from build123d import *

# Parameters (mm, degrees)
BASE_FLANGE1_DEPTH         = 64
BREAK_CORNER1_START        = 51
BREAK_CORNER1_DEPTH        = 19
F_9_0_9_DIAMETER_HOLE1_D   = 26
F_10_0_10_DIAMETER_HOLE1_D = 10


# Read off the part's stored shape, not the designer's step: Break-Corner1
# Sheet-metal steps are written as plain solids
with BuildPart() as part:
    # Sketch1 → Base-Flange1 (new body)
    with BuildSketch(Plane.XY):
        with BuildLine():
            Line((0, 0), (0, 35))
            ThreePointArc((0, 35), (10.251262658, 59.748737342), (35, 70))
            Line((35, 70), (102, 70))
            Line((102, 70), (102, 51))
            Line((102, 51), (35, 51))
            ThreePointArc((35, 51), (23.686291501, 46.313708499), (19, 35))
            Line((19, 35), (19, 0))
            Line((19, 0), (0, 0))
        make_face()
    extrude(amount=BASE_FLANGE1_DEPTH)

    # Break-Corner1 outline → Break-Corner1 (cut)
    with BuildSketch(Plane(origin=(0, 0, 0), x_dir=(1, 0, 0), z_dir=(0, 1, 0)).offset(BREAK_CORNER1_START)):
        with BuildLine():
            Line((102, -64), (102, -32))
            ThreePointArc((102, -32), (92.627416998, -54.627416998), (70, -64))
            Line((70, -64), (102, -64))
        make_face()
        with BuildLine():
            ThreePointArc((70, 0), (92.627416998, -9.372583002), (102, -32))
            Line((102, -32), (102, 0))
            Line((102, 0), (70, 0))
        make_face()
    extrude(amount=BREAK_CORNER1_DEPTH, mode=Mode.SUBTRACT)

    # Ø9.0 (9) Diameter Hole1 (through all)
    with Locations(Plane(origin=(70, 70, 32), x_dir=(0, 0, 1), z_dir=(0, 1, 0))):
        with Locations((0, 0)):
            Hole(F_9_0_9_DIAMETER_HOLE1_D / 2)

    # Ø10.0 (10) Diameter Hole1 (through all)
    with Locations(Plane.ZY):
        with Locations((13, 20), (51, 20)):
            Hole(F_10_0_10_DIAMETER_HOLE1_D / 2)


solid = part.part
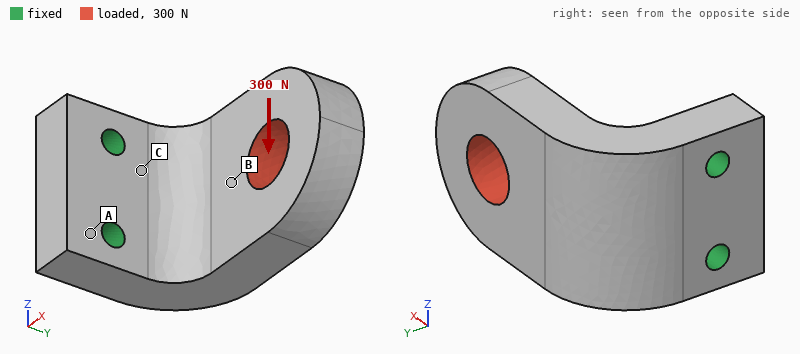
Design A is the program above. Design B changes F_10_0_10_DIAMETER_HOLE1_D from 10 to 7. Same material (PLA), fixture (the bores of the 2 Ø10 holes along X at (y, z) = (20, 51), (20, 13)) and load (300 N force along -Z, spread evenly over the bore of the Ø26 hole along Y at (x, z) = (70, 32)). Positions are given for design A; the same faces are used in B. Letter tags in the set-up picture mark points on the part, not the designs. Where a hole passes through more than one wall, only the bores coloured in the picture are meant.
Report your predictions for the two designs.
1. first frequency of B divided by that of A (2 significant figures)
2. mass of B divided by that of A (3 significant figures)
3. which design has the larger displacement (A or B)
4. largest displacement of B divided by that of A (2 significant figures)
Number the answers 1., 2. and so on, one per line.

1. 0.96
2. 1.01
3. B
4. 1.1
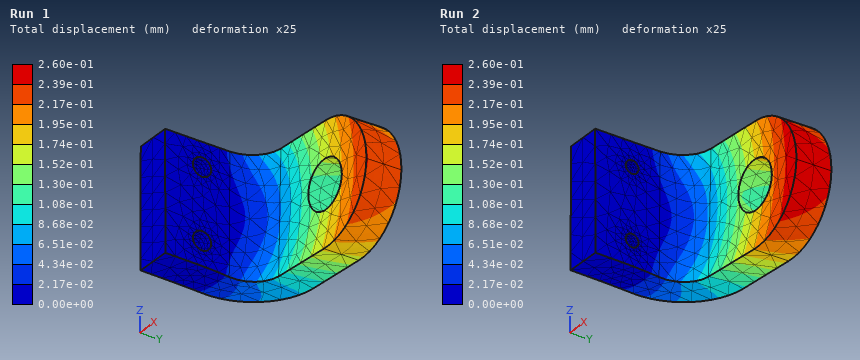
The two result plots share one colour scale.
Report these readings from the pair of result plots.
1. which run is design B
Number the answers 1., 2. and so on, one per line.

1. Run 2
